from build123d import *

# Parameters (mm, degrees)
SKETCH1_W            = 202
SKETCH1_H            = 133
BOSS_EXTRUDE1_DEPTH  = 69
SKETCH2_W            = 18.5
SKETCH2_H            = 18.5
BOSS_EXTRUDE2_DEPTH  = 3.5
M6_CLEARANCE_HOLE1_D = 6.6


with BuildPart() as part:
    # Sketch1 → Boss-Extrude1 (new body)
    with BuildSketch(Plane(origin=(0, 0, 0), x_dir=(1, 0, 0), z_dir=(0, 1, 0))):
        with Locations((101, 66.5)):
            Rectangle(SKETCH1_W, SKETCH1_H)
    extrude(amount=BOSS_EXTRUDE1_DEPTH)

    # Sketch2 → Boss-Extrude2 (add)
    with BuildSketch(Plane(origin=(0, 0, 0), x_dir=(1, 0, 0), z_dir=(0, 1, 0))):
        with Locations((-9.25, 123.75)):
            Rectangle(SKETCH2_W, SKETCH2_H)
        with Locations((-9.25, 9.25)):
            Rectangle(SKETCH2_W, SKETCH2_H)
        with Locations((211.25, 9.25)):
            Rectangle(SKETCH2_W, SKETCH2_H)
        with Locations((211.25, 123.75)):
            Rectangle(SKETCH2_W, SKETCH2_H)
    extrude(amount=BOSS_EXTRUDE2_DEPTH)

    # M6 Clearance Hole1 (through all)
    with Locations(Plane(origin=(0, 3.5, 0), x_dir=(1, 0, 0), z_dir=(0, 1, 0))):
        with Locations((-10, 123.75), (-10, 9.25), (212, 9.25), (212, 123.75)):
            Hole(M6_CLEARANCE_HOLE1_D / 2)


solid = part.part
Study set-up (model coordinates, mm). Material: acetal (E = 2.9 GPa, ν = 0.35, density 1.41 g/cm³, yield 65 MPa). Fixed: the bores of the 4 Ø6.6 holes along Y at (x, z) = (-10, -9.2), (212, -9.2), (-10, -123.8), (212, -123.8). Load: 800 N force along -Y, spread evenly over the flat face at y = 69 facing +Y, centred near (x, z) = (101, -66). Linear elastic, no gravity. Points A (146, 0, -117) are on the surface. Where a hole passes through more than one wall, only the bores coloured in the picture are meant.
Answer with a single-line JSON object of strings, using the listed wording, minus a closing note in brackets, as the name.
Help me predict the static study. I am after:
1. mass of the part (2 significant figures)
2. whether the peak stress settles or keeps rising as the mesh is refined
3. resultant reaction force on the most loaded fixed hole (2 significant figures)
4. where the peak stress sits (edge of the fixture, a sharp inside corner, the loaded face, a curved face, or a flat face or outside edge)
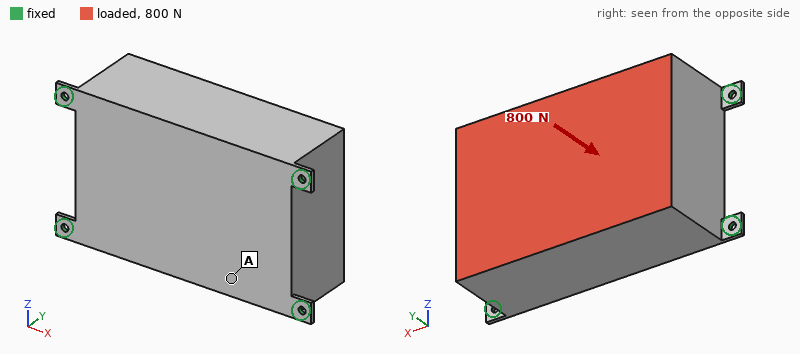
{"mass of the part": "2.6 kg", "whether the peak stress settles or keeps rising as the mesh is refined": "keeps rising", "resultant reaction force on the most loaded fixed hole": "230 N", "where the peak stress sits": "edge of the fixture"}
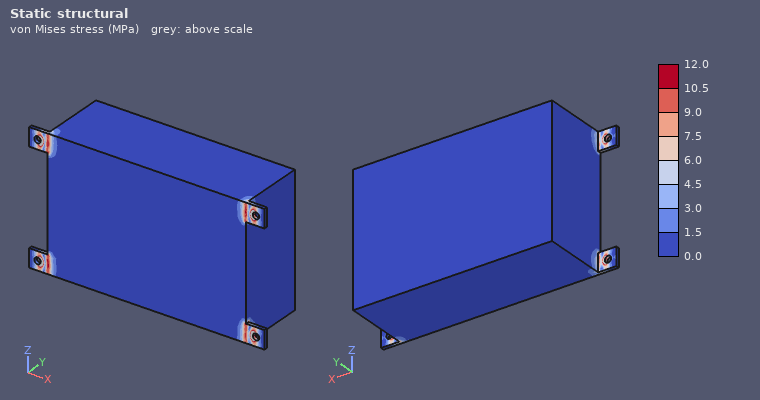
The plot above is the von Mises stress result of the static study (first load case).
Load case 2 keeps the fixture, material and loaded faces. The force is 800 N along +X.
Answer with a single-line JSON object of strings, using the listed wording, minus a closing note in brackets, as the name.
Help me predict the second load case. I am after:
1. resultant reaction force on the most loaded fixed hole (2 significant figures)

{"resultant reaction force on the most loaded fixed hole": "240 N"}
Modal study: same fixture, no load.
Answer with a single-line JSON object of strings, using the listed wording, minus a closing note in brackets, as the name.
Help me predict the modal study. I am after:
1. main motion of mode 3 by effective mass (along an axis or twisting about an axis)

{"main motion of mode 3 by effective mass": "along X"}
